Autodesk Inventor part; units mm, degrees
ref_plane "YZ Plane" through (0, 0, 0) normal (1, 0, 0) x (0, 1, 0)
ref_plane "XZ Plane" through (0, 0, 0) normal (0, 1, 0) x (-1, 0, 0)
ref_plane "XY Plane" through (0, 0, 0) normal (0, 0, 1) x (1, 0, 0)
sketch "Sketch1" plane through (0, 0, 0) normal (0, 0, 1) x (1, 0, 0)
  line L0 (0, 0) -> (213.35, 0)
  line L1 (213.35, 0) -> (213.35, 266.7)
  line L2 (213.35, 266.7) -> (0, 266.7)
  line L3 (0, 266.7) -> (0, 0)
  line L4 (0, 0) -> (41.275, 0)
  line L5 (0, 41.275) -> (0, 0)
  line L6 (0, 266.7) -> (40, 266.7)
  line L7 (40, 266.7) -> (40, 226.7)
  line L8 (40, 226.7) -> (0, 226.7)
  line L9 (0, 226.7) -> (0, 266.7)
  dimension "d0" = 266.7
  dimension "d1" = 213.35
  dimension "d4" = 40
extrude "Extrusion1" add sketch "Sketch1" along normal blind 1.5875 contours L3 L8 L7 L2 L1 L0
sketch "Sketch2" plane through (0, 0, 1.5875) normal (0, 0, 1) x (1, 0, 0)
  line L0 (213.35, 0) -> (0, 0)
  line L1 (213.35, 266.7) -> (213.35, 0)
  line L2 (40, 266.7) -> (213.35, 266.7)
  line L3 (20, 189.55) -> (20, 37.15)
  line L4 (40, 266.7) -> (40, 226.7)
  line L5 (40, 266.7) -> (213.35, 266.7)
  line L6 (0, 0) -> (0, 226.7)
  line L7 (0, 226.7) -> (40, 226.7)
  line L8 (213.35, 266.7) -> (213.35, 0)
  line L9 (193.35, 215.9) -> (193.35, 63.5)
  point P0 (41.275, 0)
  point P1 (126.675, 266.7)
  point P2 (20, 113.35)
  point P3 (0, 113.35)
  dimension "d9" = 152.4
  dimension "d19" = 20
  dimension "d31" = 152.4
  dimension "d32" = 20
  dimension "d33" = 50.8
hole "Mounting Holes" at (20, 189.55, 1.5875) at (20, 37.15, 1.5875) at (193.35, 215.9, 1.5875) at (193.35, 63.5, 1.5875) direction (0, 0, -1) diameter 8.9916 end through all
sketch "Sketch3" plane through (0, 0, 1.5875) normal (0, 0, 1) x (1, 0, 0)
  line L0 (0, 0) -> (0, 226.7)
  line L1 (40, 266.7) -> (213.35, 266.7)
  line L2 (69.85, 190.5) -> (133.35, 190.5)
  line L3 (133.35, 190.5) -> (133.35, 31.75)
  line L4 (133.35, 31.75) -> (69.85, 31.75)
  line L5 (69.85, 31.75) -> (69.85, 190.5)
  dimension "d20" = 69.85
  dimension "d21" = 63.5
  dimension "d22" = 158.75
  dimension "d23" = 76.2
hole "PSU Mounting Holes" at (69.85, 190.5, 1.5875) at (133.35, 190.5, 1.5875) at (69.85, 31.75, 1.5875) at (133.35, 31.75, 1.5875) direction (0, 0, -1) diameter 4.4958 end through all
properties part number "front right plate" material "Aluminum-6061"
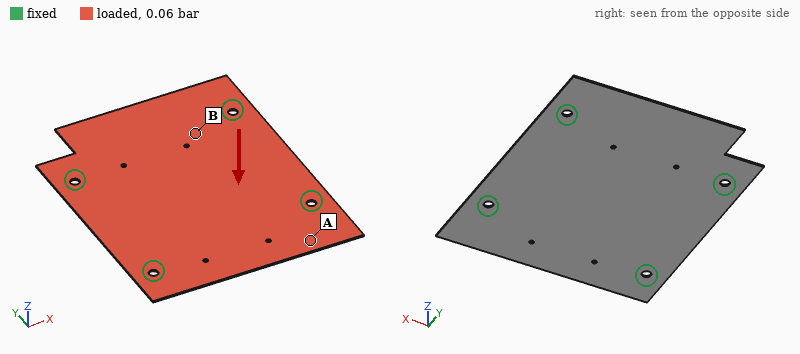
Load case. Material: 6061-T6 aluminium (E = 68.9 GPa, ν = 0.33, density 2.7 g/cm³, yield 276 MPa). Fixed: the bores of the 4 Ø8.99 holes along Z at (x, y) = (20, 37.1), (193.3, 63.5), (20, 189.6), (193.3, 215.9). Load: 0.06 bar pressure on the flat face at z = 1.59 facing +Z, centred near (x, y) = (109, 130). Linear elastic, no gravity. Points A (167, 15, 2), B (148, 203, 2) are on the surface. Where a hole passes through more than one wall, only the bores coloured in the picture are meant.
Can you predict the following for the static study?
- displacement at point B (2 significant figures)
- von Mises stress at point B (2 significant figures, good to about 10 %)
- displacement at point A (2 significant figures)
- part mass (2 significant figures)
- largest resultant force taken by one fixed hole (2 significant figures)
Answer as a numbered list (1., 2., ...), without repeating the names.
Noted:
1. 0.58 mm
2. 17 MPa
3. 0.57 mm
4. 240 g
5. 88 N
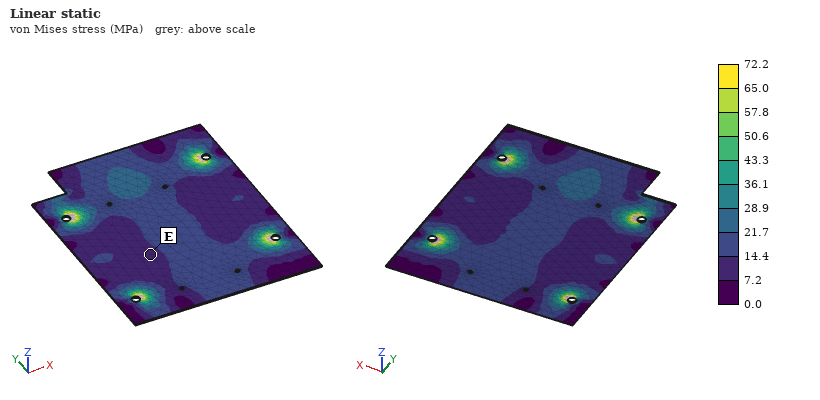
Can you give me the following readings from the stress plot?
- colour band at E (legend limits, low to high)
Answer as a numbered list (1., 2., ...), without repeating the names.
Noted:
1. 7.2 to 14.4 MPa
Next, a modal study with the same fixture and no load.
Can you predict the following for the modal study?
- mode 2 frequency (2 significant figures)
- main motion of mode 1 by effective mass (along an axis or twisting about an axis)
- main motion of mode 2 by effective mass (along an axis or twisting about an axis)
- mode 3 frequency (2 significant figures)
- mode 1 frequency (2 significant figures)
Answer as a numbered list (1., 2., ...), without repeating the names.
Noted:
1. 220 Hz
2. along Z
3. along Z
4. 250 Hz
5. 200 Hz
